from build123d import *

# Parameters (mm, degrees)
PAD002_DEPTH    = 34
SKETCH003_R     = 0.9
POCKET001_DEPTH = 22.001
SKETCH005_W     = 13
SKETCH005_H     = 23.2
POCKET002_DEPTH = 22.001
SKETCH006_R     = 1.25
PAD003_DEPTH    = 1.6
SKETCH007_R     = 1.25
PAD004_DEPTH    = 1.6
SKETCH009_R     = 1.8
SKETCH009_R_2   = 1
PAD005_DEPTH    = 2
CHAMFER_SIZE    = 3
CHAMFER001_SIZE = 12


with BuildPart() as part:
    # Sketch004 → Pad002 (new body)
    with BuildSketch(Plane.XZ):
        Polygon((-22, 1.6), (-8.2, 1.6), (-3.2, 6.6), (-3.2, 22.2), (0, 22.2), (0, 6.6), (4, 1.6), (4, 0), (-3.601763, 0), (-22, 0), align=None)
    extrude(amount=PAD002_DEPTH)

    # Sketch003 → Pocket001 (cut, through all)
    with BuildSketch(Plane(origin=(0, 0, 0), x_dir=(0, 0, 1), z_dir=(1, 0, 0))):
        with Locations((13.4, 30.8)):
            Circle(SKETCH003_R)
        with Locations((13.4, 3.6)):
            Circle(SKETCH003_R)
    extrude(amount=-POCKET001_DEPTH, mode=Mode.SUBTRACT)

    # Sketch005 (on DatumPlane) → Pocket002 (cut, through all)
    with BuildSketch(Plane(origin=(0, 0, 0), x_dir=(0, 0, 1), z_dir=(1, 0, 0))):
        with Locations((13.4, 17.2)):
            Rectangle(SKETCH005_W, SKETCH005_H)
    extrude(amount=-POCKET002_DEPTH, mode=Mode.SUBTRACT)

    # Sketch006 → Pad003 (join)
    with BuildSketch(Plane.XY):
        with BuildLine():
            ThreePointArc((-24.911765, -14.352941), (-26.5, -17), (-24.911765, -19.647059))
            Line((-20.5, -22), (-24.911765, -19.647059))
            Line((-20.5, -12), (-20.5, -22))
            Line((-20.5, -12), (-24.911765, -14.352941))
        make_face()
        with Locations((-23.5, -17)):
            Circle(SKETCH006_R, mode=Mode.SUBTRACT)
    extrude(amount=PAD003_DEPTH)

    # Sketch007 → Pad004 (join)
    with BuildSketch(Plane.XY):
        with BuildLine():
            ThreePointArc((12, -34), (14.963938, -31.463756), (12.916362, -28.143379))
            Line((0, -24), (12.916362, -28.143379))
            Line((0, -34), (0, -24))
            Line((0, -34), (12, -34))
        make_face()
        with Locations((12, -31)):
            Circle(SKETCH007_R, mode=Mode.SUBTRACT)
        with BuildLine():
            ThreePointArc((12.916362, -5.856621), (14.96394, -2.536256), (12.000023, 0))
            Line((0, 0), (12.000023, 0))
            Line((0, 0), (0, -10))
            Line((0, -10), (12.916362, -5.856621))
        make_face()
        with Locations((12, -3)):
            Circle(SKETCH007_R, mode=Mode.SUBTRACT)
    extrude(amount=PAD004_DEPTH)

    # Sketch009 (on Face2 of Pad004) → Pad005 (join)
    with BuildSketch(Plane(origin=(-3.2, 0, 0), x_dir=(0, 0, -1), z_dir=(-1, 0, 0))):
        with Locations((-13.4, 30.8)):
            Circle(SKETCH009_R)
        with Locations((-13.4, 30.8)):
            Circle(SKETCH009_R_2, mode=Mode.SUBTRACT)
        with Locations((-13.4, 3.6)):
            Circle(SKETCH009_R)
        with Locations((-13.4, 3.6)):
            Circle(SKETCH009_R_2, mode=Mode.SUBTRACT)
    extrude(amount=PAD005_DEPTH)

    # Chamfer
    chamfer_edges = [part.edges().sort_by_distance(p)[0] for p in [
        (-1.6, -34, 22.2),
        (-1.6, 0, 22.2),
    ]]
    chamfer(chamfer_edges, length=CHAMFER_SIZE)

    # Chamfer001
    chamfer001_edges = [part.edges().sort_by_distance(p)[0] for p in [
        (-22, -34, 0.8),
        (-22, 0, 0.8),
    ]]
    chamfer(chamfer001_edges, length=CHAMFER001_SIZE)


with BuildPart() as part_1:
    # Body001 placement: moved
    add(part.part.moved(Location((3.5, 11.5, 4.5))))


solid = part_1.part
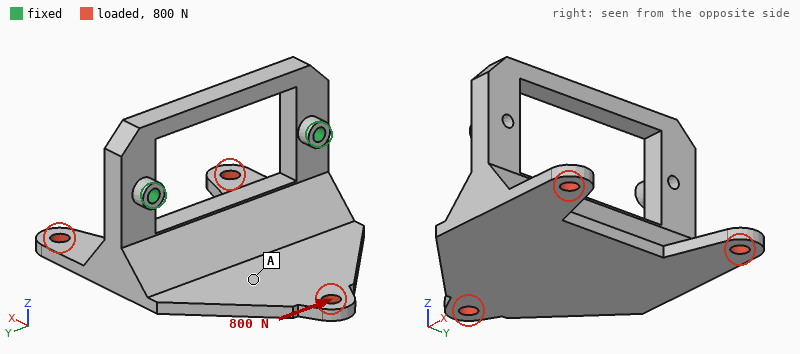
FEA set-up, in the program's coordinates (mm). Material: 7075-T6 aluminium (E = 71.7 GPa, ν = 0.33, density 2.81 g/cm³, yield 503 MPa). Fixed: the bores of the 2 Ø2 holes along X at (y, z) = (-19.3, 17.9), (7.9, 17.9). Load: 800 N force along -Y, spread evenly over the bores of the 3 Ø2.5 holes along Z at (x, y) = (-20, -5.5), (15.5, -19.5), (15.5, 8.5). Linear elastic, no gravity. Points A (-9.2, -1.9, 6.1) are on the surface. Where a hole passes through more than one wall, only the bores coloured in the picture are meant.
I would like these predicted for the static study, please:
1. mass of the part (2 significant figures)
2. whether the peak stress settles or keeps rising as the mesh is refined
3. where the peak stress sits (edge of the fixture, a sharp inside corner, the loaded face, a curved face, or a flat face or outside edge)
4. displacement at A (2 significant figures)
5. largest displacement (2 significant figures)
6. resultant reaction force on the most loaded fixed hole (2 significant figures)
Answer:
9.7 g
keeps rising
edge of the fixture
36 µm
84 µm
500 N
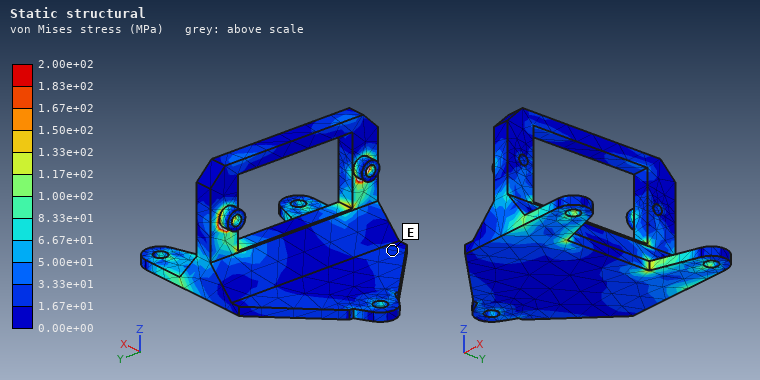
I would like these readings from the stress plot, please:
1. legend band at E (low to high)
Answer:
1.67e+01 to 3.33e+01 MPa
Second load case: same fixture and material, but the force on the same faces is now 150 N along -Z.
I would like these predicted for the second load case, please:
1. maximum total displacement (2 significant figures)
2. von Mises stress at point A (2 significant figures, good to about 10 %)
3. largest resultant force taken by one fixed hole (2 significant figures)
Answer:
0.14 mm
49 MPa
79 N
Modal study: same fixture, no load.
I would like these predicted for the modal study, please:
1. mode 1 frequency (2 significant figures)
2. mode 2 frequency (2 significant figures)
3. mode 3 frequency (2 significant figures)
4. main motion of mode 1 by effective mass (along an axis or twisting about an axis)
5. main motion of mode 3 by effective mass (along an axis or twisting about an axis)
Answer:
2100 Hz
6200 Hz
6800 Hz
along X
along Y
